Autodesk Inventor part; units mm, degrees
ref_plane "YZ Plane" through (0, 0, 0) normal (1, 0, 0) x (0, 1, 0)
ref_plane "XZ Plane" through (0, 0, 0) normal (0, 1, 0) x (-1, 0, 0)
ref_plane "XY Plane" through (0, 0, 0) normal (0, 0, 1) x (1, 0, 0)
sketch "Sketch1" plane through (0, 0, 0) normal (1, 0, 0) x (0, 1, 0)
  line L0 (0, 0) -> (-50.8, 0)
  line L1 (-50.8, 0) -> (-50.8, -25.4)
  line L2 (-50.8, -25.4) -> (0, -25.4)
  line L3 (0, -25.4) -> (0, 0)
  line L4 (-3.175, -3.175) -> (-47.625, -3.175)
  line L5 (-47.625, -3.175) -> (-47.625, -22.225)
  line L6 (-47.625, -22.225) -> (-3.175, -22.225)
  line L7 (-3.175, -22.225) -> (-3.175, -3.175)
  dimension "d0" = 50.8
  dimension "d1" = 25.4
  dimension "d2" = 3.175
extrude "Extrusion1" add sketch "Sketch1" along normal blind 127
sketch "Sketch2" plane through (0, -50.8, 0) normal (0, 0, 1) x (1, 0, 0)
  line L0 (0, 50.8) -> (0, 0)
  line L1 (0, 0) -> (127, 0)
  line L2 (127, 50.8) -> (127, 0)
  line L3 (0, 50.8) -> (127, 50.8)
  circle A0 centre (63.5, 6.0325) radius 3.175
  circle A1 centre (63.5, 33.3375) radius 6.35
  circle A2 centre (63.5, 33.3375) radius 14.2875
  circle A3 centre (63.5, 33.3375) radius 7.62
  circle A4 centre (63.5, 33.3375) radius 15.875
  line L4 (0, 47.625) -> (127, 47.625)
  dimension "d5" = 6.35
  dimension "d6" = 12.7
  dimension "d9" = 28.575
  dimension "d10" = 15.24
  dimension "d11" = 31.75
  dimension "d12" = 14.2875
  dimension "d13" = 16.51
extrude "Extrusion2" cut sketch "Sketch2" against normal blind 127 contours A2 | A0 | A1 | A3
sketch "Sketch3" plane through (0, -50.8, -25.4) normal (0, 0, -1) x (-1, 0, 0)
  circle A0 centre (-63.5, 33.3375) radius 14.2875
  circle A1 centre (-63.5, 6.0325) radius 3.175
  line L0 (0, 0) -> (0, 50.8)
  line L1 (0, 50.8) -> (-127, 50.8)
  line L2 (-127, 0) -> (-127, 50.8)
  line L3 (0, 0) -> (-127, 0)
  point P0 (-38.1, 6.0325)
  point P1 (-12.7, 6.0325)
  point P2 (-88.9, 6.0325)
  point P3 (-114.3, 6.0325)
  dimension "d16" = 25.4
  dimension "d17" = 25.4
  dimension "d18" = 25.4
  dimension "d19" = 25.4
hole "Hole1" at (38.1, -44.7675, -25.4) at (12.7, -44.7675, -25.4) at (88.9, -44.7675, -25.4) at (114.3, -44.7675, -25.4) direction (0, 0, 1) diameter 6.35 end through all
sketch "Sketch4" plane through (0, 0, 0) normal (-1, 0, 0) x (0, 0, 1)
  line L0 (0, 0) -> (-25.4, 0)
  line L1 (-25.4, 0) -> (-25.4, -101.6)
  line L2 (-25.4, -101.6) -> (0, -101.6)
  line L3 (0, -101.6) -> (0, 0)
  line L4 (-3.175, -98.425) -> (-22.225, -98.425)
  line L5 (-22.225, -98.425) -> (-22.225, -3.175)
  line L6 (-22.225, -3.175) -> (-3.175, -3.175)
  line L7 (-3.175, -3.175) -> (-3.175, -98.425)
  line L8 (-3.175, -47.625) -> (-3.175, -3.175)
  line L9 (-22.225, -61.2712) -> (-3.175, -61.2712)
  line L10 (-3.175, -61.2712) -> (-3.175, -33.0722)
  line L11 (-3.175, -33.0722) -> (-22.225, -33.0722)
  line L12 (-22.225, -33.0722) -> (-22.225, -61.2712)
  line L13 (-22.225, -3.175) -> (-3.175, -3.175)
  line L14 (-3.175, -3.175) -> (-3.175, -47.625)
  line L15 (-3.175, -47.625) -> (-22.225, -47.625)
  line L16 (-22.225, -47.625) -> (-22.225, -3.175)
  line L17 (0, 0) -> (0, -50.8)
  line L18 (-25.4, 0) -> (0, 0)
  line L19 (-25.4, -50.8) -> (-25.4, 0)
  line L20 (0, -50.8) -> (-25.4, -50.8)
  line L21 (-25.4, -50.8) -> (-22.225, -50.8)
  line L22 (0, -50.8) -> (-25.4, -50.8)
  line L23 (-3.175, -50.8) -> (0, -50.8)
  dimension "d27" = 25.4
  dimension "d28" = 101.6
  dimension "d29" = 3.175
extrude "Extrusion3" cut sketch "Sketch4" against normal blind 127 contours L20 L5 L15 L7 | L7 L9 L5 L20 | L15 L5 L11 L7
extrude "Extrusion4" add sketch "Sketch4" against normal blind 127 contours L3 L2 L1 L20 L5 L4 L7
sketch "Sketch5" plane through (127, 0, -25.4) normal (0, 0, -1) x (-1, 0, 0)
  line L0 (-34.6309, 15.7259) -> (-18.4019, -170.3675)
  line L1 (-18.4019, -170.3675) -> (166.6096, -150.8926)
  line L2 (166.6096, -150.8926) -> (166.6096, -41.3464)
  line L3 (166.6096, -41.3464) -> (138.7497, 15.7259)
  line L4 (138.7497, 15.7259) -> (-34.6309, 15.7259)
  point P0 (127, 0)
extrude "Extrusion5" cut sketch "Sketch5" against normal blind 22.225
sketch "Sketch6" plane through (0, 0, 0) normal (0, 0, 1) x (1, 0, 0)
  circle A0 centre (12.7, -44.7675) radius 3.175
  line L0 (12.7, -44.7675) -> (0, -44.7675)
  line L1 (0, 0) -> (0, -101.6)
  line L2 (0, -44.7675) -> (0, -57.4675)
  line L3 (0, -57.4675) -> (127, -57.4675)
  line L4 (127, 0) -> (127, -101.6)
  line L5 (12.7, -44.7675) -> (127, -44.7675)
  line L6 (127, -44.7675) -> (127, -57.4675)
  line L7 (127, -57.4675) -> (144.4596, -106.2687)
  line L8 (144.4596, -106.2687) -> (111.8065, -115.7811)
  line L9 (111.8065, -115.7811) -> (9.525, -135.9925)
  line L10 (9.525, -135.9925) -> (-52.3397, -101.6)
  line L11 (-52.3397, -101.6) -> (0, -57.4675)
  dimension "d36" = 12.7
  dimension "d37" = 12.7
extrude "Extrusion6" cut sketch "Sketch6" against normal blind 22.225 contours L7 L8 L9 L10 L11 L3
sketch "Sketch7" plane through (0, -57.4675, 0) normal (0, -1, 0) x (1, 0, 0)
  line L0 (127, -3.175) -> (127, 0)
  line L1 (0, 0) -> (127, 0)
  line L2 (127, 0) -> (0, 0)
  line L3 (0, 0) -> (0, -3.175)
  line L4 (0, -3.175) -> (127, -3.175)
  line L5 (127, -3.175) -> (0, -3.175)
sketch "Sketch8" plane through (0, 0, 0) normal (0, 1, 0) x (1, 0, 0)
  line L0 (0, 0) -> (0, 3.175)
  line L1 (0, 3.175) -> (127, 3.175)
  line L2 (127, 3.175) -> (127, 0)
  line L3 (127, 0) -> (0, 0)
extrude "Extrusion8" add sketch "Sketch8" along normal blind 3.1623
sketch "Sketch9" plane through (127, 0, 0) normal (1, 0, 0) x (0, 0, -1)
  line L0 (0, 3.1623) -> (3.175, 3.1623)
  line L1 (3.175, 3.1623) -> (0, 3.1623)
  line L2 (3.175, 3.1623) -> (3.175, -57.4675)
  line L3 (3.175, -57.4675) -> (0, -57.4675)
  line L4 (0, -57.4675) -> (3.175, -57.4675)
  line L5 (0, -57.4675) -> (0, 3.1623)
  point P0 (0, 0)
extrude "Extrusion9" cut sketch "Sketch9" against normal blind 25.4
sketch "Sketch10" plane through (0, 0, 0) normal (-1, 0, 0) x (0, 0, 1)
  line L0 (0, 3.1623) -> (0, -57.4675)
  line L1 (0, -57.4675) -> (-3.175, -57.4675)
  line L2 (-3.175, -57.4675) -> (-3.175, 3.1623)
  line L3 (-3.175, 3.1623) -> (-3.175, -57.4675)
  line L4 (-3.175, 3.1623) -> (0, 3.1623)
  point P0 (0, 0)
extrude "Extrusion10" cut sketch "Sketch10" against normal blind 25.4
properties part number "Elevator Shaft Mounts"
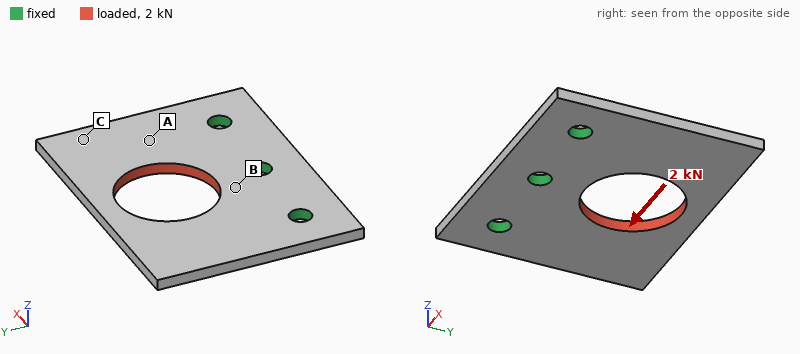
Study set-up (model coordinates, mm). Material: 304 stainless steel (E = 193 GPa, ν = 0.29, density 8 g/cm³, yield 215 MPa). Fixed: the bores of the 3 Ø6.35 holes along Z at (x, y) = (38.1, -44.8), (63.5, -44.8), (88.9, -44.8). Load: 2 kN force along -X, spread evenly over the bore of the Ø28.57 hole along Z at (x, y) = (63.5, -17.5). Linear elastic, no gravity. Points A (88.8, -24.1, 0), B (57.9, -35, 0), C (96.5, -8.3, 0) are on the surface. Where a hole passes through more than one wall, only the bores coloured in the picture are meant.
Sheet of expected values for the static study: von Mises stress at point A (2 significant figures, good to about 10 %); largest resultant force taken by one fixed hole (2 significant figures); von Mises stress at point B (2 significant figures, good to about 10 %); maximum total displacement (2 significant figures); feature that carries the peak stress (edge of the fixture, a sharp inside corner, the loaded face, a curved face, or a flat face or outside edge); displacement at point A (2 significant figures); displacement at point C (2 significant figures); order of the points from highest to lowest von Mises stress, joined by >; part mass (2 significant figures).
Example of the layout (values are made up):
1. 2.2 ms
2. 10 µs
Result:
1. 16 MPa
2. 1.1 kN
3. 31 MPa
4. 14 µm
5. edge of the fixture
6. 4.7 µm
7. 10 µm
8. B > A > C
9. 99 g
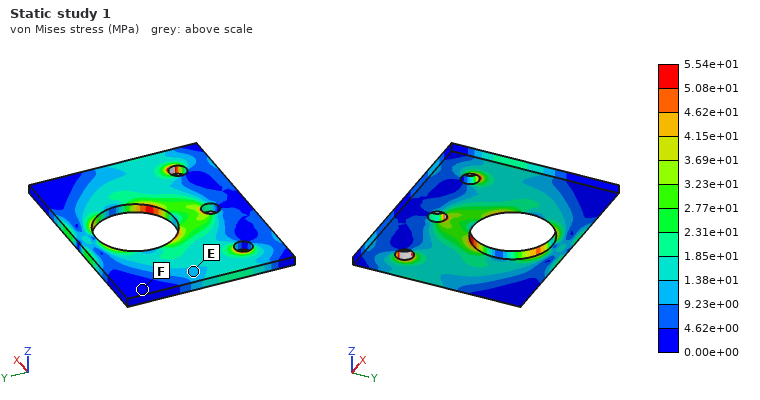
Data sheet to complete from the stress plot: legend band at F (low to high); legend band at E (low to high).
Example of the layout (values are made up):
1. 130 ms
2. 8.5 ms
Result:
1. 0.00e+00 to 4.62e+00 MPa
2. 9.23e+00 to 1.38e+01 MPa
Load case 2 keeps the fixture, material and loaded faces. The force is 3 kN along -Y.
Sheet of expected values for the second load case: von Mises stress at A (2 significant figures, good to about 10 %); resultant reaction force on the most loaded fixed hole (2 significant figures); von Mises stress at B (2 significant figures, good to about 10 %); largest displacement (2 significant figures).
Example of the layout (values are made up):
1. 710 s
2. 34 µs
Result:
1. 16 MPa
2. 1.1 kN
3. 13 MPa
4. 9.2 µm
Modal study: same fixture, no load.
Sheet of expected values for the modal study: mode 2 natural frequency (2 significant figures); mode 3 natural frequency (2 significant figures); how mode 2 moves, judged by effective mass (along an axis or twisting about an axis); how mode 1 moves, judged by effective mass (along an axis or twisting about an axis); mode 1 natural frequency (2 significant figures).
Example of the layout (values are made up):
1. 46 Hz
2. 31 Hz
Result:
1. 1800 Hz
2. 4000 Hz
3. twisting about Y
4. along Z
5. 1100 Hz
